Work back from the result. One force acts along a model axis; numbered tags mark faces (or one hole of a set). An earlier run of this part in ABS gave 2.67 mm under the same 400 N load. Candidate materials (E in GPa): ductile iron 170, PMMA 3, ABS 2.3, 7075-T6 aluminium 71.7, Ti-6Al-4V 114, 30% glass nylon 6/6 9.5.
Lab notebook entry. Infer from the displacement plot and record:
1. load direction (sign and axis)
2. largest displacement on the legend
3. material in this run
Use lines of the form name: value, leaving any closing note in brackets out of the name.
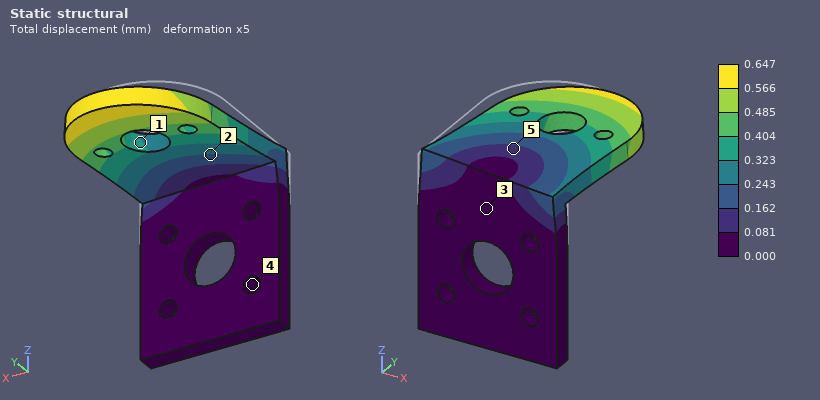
load direction: +X
largest displacement on the legend: 0.647 mm
material in this run: 30% glass nylon 6/6
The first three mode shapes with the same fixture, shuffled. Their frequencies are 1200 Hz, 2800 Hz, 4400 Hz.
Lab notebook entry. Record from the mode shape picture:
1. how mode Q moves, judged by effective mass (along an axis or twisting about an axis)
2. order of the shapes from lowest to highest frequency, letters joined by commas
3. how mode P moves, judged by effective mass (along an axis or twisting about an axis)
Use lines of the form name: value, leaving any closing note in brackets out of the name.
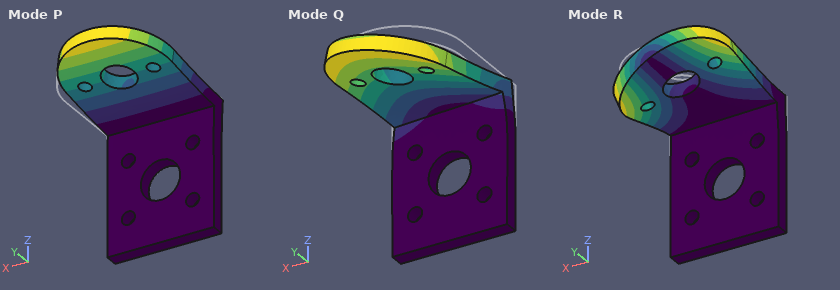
how mode Q moves, judged by effective mass: along X
order of the shapes from lowest to highest frequency, letters joined by commas: P, Q, R
how mode P moves, judged by effective mass: along Z
